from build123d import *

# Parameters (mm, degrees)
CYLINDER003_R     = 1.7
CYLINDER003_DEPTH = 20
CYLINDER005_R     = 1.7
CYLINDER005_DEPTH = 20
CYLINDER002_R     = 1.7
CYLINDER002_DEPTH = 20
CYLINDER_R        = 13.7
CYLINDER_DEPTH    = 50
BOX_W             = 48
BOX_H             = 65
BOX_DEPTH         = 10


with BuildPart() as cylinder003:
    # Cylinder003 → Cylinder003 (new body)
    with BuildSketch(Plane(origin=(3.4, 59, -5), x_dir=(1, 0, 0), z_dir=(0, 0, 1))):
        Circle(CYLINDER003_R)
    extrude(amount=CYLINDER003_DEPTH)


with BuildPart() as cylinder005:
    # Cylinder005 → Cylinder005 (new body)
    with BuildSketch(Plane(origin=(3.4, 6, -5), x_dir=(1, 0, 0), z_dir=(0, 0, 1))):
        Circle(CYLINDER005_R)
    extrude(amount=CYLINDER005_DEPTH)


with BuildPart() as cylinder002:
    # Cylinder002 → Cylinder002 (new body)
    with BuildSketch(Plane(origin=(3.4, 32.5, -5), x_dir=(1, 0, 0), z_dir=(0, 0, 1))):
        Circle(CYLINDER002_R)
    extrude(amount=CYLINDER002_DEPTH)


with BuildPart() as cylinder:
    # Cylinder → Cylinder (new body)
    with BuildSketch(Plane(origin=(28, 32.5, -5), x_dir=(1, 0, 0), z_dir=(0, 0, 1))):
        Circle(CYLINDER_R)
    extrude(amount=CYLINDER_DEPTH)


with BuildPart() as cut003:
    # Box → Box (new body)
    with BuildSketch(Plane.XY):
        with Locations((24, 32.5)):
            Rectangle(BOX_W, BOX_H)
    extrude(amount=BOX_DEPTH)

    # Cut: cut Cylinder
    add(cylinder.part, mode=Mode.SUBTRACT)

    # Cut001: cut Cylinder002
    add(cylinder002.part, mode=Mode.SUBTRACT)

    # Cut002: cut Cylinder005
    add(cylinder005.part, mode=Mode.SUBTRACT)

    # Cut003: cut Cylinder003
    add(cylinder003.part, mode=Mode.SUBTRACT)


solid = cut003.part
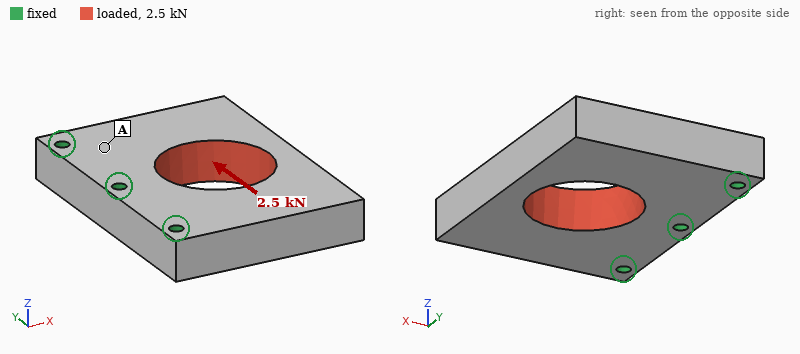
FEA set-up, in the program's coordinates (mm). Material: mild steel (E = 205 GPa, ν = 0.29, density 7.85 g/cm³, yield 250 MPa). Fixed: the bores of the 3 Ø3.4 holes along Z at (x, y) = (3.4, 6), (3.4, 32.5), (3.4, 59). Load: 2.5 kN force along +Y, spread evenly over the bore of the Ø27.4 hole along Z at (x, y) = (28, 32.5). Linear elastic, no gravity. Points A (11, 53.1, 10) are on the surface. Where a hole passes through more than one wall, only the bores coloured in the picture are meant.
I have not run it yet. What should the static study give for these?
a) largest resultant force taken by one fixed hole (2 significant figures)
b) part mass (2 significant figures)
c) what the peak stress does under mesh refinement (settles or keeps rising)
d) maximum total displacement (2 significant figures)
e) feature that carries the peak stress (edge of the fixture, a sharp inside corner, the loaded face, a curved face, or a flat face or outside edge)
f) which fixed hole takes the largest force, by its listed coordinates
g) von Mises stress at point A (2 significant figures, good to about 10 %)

1.5 kN
200 g
keeps rising
5.9 µm
edge of the fixture
(3.4, 32.5)
5.8 MPa
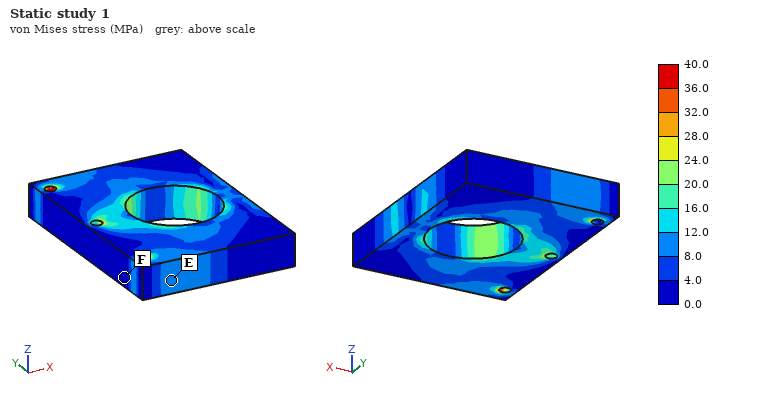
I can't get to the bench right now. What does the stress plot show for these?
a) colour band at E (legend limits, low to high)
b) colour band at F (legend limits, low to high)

8.0 to 12.0 MPa
0.0 to 4.0 MPa
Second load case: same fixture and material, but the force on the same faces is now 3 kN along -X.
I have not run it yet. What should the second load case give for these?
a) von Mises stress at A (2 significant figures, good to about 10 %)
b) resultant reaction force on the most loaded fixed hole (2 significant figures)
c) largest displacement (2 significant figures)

8.0 MPa
1.1 kN
2.9 µm
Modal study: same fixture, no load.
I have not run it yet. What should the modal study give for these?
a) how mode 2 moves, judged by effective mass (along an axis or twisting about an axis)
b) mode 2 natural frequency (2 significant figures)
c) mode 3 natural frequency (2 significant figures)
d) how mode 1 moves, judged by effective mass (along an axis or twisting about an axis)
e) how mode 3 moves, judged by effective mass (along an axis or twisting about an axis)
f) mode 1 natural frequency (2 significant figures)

twisting about X
5800 Hz
9600 Hz
along Z
along Y
3400 Hz
